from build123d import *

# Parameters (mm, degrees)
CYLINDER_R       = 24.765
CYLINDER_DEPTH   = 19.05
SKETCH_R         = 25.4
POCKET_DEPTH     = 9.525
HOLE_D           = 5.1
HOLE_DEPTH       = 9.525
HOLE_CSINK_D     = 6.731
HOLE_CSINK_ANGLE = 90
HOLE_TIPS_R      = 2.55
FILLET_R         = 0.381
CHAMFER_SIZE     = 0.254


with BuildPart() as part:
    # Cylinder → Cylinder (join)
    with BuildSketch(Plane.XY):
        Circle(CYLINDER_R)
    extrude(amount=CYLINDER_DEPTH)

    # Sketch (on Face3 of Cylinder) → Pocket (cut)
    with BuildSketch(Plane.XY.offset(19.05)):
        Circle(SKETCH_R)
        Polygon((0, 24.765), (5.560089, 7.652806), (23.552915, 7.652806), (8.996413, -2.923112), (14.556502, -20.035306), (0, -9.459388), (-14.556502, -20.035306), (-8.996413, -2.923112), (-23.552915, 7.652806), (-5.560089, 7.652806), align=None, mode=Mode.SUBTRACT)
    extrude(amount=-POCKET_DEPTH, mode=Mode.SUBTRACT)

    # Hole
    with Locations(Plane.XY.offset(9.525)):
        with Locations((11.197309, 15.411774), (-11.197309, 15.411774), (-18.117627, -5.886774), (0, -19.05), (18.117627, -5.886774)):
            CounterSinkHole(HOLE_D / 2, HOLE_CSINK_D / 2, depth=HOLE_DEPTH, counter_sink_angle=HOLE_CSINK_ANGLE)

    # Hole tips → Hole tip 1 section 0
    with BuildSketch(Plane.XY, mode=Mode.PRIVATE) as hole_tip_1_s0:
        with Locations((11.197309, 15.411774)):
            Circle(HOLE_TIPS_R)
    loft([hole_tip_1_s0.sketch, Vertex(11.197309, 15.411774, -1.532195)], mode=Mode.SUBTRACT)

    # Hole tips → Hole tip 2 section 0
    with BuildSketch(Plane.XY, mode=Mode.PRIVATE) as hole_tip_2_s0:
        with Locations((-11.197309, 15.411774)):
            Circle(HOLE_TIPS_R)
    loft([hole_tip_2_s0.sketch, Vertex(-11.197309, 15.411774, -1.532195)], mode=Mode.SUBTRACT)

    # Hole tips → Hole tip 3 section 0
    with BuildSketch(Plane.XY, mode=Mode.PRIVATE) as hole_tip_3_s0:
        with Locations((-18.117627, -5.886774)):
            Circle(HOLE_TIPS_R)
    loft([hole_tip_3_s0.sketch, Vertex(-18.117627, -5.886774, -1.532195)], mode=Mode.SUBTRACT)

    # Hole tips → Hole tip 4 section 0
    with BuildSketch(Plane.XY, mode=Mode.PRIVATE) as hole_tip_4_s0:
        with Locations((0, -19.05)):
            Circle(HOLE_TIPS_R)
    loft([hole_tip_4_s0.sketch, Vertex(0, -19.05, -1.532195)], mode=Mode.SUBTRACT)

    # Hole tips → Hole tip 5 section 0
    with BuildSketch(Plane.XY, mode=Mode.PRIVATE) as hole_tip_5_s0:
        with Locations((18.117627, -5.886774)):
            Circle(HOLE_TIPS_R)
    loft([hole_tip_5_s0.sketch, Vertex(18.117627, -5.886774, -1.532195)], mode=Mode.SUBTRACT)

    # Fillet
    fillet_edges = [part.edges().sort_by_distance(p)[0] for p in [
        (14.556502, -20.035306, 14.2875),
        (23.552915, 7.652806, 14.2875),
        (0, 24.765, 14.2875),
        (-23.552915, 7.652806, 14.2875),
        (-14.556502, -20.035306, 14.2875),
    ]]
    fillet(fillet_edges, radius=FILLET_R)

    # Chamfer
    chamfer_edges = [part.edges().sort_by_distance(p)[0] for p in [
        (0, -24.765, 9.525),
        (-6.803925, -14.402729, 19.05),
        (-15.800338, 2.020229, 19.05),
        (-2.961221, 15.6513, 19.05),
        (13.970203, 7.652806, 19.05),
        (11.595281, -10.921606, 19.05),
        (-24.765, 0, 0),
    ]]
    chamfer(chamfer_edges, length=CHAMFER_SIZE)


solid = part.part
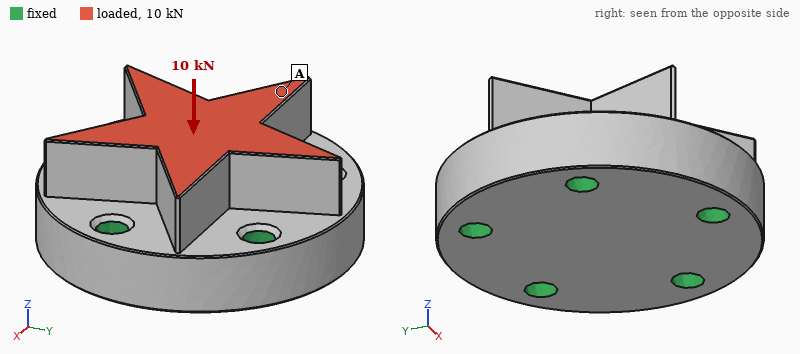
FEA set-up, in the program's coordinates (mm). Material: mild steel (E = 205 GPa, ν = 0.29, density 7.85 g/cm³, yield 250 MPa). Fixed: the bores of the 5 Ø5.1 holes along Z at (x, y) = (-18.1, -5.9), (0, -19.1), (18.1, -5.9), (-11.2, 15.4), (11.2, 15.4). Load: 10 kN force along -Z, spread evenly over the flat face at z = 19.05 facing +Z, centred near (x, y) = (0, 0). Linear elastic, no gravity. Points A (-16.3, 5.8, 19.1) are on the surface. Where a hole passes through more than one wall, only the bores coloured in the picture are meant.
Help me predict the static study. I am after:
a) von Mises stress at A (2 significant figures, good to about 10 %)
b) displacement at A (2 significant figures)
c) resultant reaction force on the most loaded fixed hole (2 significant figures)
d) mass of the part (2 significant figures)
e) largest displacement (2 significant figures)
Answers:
13 MPa
2.0 µm
2.1 kN
190 g
2.6 µm
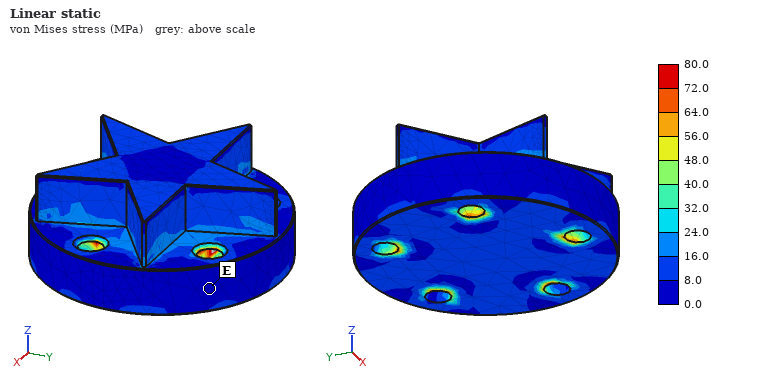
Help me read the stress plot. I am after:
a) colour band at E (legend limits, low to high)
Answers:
0.0 to 8.0 MPa
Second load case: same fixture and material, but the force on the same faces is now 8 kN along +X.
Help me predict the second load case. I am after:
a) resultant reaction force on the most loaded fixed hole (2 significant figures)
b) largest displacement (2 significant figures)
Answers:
3.0 kN
7.7 µm
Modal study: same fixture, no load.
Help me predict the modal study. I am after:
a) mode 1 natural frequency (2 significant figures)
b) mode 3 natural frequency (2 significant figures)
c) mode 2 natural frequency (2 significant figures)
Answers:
35 kHz
36 kHz
36 kHz
